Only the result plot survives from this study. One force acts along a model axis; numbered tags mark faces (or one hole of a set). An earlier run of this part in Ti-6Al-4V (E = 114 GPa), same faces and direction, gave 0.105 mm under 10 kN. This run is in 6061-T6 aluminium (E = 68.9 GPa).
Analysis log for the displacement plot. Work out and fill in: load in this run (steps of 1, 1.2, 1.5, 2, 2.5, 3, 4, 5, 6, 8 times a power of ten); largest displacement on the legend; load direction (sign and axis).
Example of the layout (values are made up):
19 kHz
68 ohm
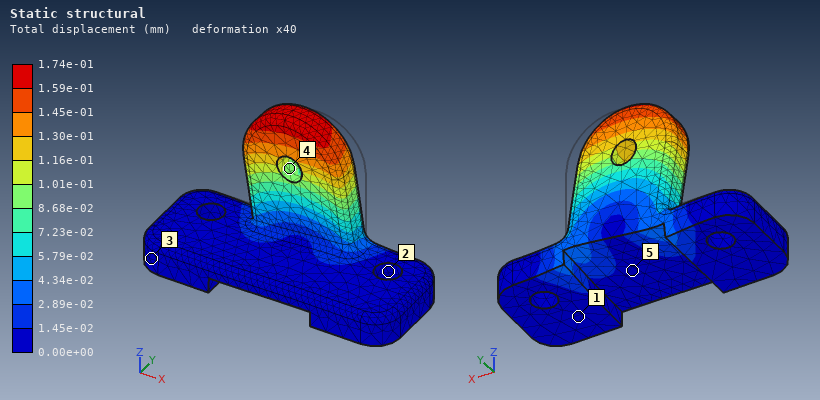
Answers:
10 kN
1.74e-01 mm
-X
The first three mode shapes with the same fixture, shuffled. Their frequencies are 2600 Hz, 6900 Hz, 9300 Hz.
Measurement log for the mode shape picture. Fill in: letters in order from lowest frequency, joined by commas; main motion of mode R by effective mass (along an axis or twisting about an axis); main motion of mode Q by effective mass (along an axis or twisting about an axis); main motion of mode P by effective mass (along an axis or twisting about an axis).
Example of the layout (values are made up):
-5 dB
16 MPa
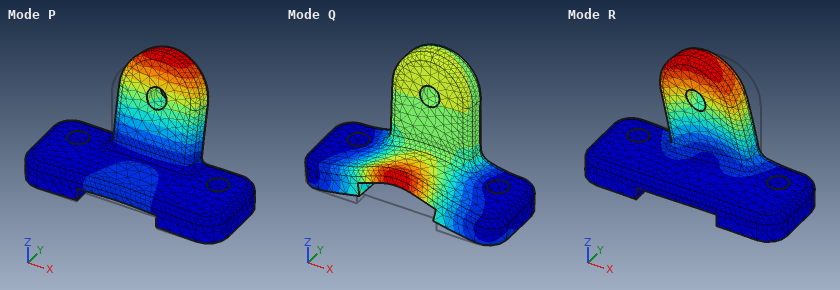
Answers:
P, R, Q
along X
along Z
along Y
